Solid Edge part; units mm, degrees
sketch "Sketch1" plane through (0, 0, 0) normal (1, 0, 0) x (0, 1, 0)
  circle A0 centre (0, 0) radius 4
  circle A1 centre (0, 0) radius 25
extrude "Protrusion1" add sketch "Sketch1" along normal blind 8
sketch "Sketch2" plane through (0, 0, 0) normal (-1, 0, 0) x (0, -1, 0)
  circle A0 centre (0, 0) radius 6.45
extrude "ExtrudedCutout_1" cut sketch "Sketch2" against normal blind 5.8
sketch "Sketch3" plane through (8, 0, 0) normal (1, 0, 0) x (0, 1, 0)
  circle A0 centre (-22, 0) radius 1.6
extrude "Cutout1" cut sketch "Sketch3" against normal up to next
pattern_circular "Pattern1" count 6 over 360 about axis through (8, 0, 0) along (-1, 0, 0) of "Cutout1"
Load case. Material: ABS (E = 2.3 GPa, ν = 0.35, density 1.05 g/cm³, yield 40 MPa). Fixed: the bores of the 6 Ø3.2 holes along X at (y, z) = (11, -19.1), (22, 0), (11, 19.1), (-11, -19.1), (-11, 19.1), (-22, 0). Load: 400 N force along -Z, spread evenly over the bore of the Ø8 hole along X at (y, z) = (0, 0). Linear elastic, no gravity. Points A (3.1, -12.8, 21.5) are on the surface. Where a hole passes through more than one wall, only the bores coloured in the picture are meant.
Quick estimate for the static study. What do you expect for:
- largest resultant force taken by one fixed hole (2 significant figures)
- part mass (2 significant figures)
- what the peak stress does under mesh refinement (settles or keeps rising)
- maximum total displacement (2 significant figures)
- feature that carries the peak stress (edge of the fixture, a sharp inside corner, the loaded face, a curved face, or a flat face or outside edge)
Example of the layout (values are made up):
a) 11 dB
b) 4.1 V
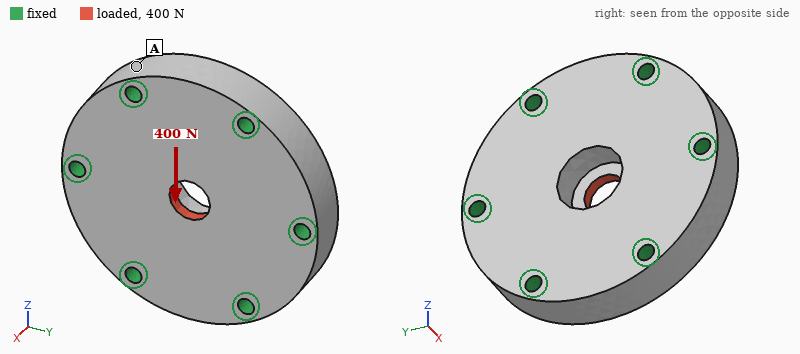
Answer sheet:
a) 93 N
b) 15 g
c) keeps rising
d) 30 µm
e) a sharp inside corner
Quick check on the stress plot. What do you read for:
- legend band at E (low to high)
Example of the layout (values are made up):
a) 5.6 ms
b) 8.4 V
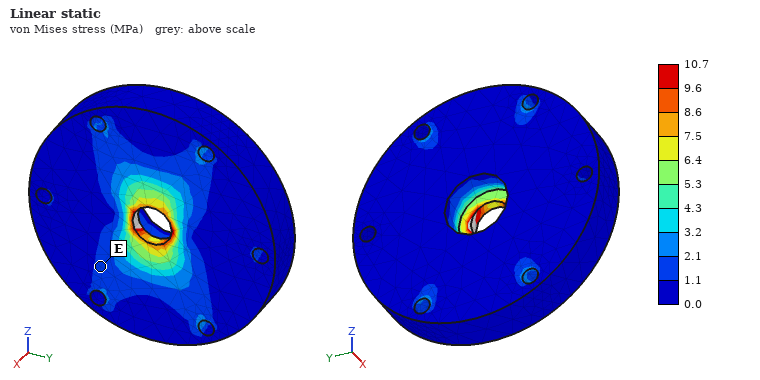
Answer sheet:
a) 1.1 to 2.1 MPa
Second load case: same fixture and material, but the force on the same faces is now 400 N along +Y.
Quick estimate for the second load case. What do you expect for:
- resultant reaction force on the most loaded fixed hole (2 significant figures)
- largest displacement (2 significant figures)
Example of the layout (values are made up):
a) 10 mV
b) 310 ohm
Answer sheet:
a) 110 N
b) 30 µm
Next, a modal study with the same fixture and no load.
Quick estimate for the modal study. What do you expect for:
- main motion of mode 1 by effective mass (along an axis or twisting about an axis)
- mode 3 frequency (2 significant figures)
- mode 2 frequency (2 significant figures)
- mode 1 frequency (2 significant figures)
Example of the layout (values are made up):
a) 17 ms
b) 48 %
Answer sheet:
a) along X
b) 12 kHz
c) 12 kHz
d) 8000 Hz
